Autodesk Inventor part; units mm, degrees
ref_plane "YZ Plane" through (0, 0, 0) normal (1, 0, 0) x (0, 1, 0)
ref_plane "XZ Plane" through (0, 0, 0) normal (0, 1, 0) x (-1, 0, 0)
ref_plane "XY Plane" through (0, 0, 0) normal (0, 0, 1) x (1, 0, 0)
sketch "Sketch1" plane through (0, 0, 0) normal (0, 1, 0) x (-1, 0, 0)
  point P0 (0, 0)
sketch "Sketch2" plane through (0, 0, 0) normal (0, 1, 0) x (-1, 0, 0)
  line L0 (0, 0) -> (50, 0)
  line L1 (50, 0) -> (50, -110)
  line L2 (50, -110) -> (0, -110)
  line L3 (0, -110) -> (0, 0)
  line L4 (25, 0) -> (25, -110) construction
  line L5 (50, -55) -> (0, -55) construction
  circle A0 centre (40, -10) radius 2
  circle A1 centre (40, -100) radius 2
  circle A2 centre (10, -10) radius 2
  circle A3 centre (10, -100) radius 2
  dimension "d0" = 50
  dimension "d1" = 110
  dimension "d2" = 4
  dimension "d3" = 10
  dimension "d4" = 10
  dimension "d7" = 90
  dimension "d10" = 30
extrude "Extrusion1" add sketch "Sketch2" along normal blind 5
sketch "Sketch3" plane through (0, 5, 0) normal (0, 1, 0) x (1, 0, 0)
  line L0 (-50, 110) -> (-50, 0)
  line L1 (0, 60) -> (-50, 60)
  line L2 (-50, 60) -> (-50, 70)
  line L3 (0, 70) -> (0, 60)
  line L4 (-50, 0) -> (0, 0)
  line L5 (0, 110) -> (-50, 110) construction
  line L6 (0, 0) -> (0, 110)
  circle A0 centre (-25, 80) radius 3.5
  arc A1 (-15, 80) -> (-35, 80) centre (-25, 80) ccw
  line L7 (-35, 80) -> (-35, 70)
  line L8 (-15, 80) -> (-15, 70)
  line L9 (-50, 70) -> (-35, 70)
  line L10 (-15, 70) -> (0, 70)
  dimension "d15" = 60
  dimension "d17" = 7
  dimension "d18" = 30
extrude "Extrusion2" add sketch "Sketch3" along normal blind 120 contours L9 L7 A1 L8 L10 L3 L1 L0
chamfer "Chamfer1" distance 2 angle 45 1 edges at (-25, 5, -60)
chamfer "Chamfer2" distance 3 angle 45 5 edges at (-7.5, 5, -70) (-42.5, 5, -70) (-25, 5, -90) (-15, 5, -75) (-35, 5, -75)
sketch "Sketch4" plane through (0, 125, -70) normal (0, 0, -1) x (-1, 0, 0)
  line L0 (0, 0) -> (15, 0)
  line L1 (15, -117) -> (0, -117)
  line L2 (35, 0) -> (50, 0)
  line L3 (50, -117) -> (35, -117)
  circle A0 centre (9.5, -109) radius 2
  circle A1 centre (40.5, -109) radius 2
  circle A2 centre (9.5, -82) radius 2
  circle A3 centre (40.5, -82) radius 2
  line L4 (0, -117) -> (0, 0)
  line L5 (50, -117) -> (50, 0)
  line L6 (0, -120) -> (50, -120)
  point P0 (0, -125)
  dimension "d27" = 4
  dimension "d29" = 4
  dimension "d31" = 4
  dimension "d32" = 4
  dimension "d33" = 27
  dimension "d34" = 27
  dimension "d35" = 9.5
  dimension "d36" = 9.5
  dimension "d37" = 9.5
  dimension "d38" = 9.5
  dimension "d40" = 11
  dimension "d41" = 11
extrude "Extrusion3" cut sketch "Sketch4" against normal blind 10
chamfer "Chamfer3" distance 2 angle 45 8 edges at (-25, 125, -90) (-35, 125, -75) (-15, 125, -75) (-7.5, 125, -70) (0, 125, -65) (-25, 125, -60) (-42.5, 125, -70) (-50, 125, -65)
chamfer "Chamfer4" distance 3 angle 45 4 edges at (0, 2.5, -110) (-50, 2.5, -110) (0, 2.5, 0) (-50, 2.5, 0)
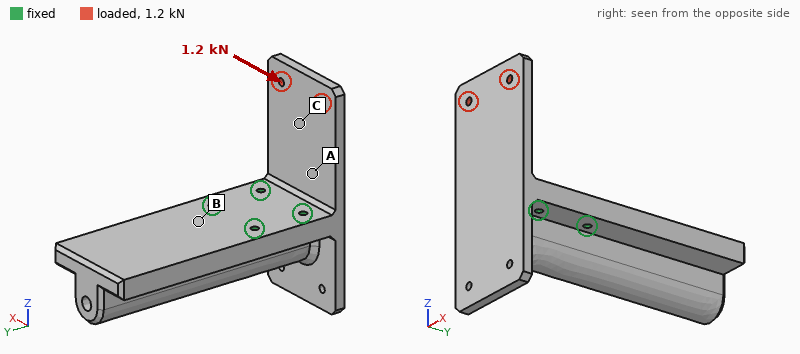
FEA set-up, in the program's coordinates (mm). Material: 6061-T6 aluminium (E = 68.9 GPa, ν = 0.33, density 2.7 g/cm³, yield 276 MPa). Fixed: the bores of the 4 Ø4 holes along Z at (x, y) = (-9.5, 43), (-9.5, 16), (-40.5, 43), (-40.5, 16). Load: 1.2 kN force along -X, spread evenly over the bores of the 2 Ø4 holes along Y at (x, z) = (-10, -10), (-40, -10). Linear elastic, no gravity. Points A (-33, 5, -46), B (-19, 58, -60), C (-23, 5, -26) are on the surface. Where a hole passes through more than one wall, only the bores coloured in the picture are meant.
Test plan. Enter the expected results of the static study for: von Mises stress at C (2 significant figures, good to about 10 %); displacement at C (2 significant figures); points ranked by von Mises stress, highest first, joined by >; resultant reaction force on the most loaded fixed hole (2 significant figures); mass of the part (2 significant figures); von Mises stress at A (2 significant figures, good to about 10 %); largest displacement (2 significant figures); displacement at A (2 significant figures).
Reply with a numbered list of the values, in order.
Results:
1. 13 MPa
2. 41 µm
3. A > C > B
4. 1.9 kN
5. 340 g
6. 16 MPa
7. 76 µm
8. 19 µm
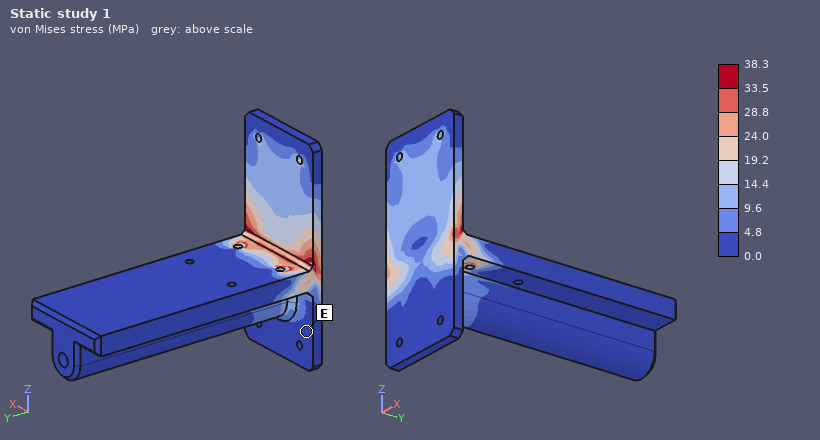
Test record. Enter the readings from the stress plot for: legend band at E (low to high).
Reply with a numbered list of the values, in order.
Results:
1. 0.0 to 4.8 MPa
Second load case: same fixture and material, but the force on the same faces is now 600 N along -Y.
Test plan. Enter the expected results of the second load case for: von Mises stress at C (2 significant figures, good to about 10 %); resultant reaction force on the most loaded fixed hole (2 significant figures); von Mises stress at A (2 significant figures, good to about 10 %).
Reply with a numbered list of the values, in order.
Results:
1. 41 MPa
2. 750 N
3. 94 MPa
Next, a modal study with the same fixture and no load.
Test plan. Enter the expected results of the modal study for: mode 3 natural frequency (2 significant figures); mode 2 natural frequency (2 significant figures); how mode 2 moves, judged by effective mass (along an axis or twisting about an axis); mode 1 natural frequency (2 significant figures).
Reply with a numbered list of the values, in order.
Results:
1. 3000 Hz
2. 2100 Hz
3. along Z
4. 1100 Hz
